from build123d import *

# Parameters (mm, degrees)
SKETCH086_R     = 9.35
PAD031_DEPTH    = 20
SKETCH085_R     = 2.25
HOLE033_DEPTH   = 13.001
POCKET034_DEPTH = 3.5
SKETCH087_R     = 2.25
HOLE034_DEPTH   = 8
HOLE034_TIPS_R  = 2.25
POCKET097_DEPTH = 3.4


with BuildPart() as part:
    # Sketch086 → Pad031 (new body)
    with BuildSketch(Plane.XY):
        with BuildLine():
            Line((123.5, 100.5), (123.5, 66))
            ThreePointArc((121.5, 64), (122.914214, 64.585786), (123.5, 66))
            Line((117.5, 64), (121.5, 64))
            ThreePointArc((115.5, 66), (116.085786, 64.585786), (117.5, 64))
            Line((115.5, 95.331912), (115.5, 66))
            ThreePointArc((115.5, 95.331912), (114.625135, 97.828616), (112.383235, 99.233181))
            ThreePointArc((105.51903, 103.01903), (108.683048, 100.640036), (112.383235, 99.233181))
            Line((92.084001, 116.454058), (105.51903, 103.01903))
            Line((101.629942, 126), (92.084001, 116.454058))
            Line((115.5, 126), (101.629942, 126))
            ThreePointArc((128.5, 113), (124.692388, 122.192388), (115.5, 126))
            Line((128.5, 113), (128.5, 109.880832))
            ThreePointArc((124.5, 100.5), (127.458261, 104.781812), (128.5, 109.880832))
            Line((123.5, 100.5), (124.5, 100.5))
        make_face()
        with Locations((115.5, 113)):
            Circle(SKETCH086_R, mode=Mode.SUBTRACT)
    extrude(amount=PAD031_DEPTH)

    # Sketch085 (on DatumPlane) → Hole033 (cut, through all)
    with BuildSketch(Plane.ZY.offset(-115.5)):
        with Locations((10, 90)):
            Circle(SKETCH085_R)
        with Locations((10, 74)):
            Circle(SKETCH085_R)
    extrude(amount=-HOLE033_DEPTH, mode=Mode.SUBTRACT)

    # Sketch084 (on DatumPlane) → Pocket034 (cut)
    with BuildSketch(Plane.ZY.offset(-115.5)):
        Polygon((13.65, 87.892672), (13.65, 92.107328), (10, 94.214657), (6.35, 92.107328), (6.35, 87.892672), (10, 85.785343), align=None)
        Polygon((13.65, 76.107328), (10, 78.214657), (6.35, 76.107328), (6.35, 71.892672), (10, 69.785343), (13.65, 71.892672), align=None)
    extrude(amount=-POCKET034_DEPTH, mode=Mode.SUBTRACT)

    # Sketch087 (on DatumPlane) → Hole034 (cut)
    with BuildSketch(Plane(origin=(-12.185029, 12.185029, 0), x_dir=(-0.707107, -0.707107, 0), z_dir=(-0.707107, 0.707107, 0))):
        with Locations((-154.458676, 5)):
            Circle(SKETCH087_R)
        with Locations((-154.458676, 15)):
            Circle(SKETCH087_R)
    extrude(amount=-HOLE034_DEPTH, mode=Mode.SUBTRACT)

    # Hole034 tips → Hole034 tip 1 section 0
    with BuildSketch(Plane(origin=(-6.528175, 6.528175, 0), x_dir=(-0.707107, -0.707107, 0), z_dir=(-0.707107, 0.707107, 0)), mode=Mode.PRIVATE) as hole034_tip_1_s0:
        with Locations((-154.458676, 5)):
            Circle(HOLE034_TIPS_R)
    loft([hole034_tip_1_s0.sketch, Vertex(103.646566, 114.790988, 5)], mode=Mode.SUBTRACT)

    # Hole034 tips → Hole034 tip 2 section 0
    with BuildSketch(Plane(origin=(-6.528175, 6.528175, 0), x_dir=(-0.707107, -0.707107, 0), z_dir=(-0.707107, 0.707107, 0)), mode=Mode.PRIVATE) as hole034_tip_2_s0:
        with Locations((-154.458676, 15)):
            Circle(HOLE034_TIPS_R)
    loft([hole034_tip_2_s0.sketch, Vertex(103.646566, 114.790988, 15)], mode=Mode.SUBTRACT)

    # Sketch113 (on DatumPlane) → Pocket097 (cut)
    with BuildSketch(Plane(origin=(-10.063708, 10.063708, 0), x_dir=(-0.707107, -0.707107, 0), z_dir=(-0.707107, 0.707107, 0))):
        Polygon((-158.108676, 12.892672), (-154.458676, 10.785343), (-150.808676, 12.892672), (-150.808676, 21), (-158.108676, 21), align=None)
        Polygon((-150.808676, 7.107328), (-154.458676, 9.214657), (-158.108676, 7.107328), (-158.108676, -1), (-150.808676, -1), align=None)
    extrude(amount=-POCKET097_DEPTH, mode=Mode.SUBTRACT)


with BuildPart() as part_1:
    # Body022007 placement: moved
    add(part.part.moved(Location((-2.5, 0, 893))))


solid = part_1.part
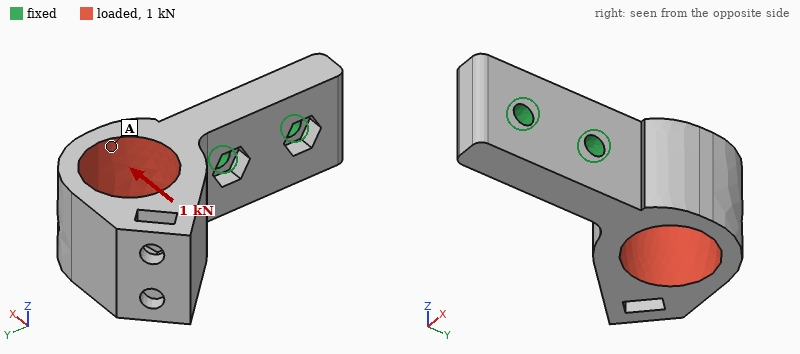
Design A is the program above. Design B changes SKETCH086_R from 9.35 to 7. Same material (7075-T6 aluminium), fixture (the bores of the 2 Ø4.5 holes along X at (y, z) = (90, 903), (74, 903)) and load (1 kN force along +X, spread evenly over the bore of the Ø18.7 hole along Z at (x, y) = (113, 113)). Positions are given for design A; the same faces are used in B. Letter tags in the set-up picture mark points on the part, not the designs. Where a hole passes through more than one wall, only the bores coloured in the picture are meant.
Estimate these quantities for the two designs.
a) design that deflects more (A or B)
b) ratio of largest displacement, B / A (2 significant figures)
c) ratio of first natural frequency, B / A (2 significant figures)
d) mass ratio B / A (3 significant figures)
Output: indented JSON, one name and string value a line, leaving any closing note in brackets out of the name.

{
  "design that deflects more": "A",
  "ratio of largest displacement, B / A": "0.86",
  "ratio of first natural frequency, B / A": "0.98",
  "mass ratio B / A": "1.18"
}
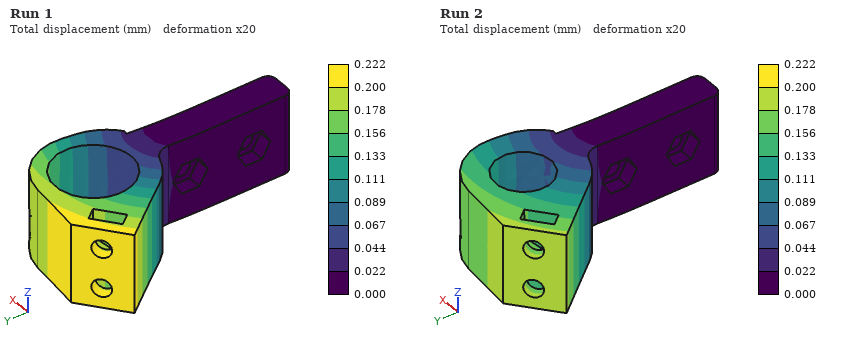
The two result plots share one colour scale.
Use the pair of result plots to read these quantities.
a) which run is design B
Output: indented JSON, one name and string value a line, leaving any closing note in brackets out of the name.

{
  "which run is design B": "Run 2"
}
